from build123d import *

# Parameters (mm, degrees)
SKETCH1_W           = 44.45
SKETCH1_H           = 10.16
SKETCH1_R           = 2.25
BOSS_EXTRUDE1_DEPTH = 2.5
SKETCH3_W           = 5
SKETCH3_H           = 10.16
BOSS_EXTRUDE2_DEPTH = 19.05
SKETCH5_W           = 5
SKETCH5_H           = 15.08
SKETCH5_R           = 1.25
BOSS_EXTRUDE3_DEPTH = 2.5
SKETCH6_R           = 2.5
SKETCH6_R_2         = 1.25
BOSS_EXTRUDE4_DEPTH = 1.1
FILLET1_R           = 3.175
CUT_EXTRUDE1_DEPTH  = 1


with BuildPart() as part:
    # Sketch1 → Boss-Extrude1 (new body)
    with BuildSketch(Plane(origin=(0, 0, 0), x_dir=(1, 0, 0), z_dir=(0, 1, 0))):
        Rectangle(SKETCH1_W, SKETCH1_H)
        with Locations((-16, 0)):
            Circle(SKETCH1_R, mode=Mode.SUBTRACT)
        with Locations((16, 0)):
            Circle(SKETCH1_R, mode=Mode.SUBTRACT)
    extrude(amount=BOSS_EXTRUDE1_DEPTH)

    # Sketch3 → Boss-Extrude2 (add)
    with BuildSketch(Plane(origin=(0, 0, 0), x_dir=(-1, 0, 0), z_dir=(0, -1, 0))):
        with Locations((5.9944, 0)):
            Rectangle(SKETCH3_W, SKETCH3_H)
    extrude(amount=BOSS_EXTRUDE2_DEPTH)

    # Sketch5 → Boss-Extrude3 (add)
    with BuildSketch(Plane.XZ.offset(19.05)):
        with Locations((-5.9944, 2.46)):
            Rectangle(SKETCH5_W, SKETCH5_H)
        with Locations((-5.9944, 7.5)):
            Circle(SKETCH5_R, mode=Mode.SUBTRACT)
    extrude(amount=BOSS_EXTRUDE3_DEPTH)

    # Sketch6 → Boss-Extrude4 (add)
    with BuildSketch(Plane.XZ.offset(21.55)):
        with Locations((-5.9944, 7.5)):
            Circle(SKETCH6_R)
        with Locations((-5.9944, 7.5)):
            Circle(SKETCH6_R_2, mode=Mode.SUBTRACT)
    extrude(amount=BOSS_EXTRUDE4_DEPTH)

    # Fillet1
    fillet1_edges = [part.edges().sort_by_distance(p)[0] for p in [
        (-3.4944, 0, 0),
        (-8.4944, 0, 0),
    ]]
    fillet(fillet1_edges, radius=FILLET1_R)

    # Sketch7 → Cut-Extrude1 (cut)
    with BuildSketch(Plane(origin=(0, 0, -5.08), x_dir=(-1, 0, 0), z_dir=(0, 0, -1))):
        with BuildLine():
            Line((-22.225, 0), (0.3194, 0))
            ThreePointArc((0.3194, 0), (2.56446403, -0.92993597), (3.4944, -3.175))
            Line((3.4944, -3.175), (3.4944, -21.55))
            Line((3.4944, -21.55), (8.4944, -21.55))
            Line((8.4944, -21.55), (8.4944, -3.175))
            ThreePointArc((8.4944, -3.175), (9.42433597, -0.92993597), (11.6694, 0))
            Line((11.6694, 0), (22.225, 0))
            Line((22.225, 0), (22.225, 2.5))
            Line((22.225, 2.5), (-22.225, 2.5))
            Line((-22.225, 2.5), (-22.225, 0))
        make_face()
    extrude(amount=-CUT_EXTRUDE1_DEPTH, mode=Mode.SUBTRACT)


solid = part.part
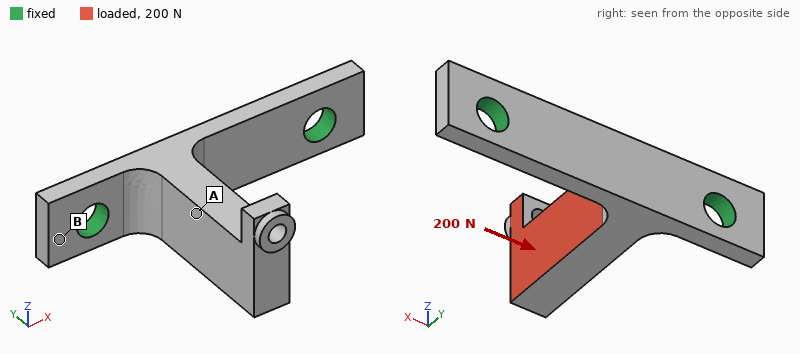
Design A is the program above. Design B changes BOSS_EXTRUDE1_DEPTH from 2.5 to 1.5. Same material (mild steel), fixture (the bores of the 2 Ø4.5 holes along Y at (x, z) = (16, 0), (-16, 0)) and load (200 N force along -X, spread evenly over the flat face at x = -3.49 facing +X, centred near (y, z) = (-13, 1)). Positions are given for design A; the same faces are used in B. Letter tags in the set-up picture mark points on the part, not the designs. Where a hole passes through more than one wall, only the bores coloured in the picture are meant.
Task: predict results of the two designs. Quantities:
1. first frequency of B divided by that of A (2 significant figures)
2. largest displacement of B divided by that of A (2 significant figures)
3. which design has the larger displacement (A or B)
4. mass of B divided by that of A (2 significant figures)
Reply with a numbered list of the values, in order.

1. 0.59
2. 2.7
3. B
4. 0.82
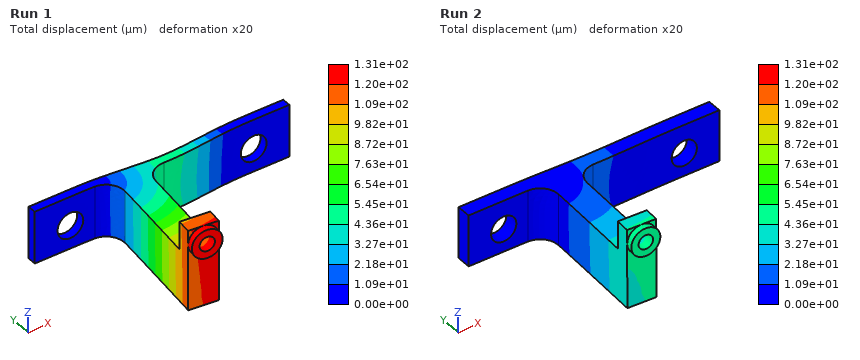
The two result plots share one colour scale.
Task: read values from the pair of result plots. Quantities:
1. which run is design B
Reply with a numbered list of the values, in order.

1. Run 1
